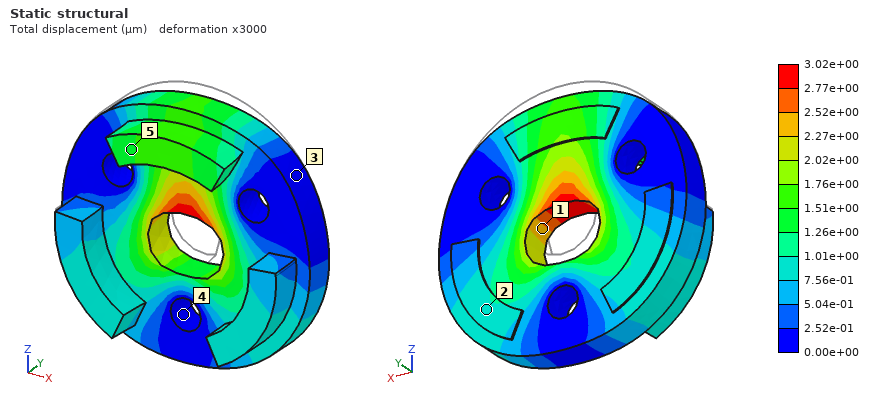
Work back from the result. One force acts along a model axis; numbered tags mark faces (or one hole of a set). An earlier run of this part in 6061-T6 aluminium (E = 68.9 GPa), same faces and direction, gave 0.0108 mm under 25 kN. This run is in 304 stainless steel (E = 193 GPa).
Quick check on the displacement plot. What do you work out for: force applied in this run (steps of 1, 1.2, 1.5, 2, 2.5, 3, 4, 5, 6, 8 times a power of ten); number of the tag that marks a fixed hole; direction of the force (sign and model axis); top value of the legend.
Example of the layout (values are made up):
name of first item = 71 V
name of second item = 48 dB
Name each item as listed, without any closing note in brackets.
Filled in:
force applied in this run = 20 kN
number of the tag that marks a fixed hole = 4
direction of the force = -Z
top value of the legend = 3.02e+00 µm
